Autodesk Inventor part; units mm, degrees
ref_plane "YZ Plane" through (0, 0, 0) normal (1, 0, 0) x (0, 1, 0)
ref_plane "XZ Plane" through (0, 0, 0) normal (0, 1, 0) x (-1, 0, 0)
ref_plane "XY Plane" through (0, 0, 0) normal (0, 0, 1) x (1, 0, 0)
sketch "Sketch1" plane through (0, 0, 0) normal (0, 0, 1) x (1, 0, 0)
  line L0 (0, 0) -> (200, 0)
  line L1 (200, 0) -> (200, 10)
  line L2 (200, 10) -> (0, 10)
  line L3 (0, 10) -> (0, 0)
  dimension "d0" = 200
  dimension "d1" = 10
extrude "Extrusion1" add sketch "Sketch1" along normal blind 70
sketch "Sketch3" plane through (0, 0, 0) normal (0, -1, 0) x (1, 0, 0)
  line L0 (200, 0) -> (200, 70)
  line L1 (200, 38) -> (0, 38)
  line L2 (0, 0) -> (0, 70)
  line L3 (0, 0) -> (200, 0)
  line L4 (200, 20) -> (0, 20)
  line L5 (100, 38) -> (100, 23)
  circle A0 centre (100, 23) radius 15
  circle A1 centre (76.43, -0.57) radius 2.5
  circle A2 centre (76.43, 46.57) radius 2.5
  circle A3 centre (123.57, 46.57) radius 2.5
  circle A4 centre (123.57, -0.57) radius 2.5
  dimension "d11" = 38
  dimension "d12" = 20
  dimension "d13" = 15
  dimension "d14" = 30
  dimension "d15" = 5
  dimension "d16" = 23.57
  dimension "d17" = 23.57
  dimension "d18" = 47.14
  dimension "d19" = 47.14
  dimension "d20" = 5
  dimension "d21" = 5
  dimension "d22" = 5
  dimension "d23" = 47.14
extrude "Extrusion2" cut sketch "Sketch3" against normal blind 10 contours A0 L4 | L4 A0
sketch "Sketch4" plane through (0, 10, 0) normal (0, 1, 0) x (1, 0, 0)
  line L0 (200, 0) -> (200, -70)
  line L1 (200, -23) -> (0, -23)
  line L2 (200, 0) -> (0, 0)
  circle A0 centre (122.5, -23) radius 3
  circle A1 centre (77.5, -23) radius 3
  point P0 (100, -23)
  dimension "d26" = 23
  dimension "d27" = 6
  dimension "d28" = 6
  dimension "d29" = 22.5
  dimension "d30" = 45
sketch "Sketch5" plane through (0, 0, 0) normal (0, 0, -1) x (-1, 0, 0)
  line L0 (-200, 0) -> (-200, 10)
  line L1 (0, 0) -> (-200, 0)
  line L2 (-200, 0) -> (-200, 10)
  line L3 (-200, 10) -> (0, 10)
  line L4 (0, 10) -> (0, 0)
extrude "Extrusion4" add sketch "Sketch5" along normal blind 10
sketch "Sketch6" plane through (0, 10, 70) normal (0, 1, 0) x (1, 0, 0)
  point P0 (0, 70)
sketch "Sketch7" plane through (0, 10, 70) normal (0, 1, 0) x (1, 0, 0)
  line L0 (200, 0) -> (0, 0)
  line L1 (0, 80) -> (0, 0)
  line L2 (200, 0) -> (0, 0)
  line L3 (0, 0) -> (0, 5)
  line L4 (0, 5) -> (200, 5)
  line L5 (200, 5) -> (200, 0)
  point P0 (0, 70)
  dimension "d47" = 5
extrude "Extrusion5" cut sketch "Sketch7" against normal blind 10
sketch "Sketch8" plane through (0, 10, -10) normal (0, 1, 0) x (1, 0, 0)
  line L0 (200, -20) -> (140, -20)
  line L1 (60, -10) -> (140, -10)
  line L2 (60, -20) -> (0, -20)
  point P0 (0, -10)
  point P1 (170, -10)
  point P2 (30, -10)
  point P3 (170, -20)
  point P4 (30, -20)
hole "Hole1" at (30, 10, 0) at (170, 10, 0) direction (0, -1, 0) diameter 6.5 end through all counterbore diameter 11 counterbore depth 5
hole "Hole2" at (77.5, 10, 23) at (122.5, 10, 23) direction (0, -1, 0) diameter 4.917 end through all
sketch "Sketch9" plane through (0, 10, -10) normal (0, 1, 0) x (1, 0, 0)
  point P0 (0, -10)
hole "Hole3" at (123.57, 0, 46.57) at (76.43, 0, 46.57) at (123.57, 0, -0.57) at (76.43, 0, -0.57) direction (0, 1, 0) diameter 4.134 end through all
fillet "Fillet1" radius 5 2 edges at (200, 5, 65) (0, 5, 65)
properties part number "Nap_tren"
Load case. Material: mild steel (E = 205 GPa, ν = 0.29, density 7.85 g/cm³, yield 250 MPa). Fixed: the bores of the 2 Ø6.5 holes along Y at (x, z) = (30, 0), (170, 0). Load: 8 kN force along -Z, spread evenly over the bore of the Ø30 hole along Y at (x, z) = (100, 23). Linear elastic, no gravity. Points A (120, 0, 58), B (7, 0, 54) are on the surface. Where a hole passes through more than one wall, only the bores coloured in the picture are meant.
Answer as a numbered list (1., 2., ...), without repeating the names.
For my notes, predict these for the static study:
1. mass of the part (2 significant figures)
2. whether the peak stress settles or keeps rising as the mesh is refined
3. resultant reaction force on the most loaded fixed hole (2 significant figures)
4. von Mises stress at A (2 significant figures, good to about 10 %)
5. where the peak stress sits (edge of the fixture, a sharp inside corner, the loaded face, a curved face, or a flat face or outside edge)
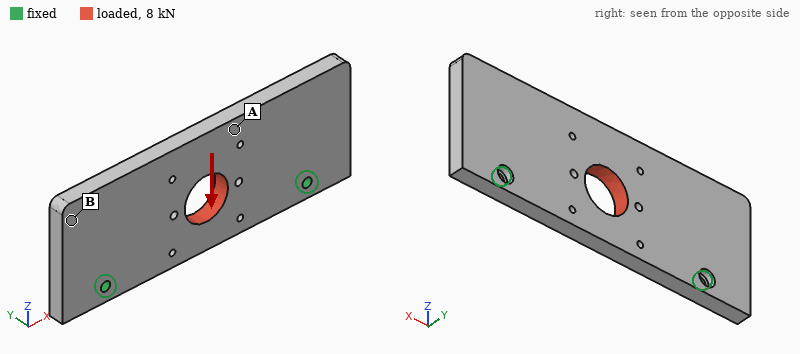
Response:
1. 1.1 kg
2. keeps rising
3. 4.6 kN
4. 19 MPa
5. edge of the fixture
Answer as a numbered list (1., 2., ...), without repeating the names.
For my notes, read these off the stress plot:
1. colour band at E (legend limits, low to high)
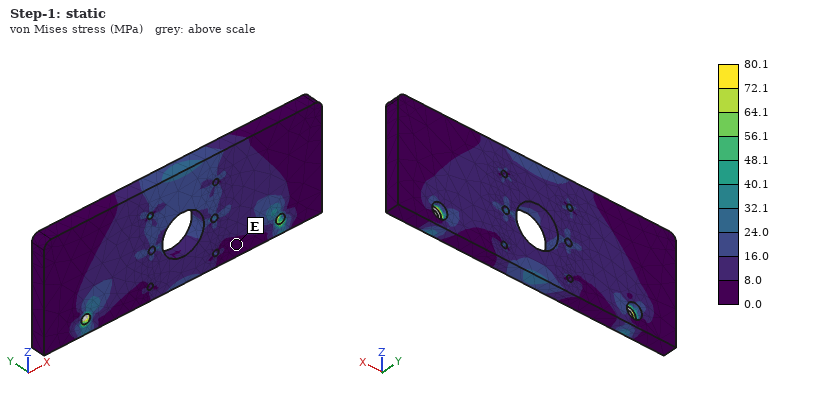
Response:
1. 0.0 to 8.0 MPa
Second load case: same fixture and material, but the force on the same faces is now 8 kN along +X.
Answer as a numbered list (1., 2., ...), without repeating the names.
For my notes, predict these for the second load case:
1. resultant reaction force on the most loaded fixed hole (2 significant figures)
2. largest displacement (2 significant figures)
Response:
1. 4.2 kN
2. 7.4 µm
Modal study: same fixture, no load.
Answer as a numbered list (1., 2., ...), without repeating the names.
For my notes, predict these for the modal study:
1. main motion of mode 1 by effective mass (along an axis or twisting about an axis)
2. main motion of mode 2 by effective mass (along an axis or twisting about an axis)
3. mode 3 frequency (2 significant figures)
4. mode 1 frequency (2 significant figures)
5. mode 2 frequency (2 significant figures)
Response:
1. along Y
2. twisting about Z
3. 1800 Hz
4. 840 Hz
5. 1600 Hz
